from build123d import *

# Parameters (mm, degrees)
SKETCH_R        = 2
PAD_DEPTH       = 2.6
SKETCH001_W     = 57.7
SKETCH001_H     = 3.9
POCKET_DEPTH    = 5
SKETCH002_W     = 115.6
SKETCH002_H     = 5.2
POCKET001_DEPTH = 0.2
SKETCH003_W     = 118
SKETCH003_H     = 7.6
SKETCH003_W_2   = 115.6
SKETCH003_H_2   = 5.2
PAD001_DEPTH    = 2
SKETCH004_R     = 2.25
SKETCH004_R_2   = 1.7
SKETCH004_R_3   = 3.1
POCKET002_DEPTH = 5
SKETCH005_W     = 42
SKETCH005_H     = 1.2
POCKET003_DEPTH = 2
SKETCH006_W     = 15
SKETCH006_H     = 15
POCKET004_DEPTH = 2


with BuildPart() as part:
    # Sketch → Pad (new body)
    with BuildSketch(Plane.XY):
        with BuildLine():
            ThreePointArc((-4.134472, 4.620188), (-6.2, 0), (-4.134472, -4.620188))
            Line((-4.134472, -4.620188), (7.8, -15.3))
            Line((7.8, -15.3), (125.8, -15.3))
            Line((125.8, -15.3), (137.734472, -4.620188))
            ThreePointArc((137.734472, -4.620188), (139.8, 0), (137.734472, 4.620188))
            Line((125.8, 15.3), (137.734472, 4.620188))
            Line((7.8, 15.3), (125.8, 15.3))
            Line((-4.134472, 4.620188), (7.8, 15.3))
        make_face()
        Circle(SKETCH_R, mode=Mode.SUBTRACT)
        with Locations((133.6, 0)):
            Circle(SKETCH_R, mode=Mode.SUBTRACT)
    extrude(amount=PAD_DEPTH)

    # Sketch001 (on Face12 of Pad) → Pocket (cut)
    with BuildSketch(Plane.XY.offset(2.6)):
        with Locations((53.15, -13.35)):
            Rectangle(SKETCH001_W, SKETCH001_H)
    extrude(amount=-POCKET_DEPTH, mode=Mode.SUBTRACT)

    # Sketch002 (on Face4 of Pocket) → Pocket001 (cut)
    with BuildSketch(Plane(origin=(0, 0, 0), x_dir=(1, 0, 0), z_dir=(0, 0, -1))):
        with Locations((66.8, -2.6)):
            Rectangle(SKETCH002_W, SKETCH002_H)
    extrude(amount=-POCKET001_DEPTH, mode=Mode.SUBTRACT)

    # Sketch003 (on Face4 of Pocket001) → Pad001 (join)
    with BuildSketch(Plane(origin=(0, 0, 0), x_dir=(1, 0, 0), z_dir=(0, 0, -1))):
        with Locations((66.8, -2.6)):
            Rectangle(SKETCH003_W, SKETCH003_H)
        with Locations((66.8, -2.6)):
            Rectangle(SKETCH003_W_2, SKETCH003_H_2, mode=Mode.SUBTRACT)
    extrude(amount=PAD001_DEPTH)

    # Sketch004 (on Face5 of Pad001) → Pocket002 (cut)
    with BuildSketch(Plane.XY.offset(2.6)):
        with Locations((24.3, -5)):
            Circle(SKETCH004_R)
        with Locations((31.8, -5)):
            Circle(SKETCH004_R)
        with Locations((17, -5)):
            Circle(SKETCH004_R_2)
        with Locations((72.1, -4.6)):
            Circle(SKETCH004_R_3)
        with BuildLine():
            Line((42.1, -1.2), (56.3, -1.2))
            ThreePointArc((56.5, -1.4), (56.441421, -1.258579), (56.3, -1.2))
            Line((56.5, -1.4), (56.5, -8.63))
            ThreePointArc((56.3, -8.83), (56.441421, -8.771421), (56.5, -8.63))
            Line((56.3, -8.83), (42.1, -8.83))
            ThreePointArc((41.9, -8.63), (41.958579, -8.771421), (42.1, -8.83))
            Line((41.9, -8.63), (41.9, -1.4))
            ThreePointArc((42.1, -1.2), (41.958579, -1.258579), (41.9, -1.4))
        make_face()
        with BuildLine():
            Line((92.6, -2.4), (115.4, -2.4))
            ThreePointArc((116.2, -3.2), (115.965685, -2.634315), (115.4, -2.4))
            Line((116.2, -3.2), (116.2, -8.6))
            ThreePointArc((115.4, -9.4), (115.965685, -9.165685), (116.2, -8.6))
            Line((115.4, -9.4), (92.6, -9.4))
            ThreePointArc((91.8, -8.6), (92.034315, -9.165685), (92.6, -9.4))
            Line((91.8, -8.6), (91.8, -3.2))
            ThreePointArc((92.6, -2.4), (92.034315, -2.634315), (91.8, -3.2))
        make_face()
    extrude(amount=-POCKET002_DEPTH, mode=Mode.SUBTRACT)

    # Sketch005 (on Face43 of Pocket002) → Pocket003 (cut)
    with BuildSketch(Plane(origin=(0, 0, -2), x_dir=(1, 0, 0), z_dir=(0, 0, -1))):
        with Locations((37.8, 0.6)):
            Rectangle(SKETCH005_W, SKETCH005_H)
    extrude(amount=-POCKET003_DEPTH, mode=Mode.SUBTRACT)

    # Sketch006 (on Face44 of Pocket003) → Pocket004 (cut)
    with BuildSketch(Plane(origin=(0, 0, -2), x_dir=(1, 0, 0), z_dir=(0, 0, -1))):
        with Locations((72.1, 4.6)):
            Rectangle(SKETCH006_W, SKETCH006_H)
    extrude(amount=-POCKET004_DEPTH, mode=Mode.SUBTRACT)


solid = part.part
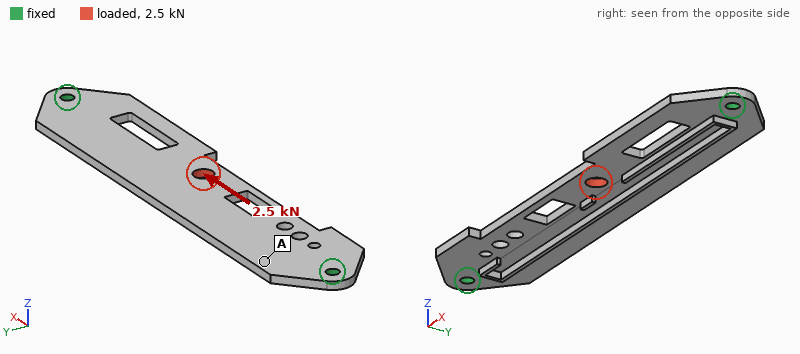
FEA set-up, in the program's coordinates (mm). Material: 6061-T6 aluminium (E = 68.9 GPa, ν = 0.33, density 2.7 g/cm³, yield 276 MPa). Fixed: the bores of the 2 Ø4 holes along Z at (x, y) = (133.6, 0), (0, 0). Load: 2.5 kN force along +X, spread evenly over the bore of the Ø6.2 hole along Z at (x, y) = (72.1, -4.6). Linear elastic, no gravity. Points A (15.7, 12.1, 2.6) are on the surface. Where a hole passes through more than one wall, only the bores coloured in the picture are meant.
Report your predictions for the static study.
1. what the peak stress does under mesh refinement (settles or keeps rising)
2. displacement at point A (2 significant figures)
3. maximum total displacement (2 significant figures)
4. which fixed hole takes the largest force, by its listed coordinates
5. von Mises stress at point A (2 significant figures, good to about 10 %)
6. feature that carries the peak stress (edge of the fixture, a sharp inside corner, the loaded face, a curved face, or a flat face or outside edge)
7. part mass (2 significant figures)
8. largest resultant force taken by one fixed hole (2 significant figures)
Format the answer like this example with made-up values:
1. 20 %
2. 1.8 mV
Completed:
1. keeps rising
2. 17 µm
3. 37 µm
4. (133.6, 0)
5. 9.5 MPa
6. a sharp inside corner
7. 26 g
8. 1.5 kN
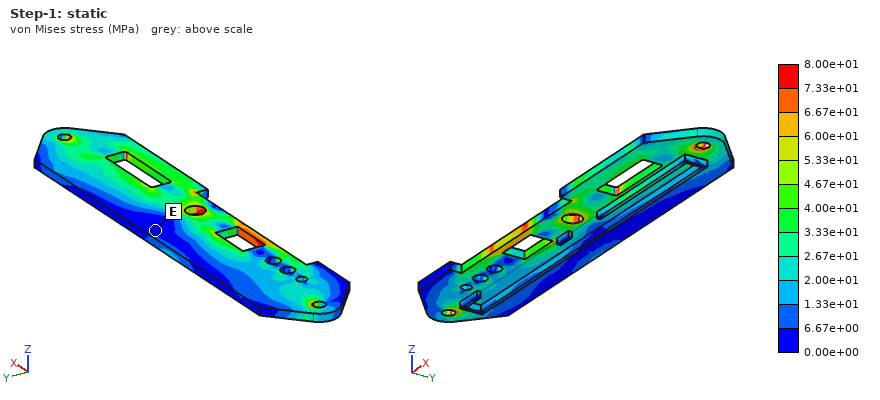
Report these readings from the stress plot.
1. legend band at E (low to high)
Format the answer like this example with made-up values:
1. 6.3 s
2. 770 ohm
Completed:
1. 0.00e+00 to 6.67e+00 MPa
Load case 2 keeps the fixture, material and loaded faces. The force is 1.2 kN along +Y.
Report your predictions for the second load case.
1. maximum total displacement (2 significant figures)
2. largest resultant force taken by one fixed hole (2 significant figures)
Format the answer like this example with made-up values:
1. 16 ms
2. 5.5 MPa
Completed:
1. 0.19 mm
2. 860 N
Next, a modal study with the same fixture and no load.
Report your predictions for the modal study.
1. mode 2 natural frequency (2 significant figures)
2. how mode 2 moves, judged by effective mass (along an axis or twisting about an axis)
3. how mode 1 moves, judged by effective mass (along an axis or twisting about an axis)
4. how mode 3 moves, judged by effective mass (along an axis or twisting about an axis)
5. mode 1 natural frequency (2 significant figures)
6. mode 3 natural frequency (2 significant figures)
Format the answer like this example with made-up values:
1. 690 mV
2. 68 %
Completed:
1. 1900 Hz
2. twisting about X
3. along Z
4. twisting about Y
5. 790 Hz
6. 2200 Hz
